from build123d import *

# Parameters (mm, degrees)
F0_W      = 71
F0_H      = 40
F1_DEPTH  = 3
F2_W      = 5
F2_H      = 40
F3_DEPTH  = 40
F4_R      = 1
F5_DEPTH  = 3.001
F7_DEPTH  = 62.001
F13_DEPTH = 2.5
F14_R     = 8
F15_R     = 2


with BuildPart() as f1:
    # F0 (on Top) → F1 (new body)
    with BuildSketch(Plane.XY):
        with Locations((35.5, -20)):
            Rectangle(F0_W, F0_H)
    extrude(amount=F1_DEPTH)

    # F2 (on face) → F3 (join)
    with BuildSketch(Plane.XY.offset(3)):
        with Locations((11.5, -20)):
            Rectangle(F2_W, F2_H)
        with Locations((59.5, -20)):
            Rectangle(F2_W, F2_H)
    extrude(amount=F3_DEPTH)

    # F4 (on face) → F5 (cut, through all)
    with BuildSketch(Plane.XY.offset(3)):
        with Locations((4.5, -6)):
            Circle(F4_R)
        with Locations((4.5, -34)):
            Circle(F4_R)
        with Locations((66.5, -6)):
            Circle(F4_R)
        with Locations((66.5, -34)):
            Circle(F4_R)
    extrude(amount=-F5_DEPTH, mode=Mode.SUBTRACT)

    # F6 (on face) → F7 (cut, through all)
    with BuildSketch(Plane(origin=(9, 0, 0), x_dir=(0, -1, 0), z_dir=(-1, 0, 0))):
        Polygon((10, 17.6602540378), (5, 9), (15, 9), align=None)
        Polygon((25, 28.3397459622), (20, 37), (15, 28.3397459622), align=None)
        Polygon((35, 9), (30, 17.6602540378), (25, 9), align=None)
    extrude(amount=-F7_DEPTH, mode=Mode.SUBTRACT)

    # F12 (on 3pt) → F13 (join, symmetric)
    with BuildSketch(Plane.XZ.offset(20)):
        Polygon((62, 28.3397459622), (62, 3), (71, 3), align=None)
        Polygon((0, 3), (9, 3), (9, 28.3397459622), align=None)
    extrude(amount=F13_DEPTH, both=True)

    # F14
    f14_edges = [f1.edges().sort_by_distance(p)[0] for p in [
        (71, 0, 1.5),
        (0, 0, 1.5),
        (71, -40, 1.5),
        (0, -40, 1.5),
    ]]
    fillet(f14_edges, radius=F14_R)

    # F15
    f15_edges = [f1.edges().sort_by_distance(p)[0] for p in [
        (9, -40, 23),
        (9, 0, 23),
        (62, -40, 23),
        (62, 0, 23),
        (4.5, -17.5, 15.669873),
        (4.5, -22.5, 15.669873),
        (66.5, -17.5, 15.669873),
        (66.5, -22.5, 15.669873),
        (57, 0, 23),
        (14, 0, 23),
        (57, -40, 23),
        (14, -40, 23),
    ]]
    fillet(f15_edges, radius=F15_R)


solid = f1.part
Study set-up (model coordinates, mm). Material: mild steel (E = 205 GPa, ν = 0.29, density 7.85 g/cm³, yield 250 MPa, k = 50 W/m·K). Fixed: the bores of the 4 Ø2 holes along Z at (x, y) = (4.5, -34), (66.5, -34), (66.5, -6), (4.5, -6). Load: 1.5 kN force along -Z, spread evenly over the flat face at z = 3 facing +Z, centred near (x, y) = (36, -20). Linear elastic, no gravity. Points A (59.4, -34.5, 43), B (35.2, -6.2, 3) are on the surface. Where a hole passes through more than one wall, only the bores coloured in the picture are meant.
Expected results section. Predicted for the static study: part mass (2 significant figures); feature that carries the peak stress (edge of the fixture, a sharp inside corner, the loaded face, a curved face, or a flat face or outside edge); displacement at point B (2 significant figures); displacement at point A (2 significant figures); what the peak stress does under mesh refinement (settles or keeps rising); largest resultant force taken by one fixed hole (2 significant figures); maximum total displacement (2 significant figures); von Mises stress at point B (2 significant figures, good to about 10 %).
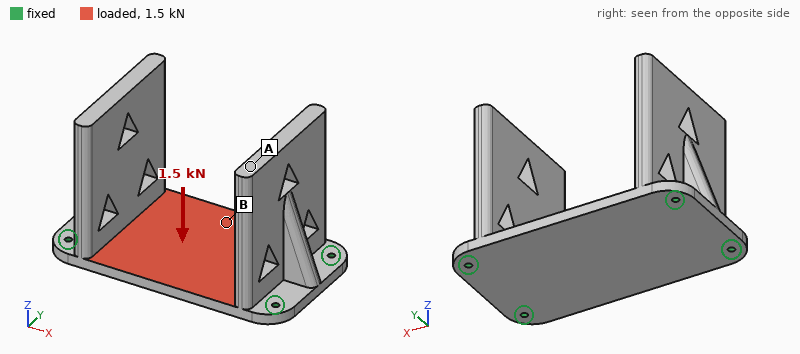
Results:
190 g
edge of the fixture
0.082 mm
0.13 mm
keeps rising
380 N
0.14 mm
92 MPa
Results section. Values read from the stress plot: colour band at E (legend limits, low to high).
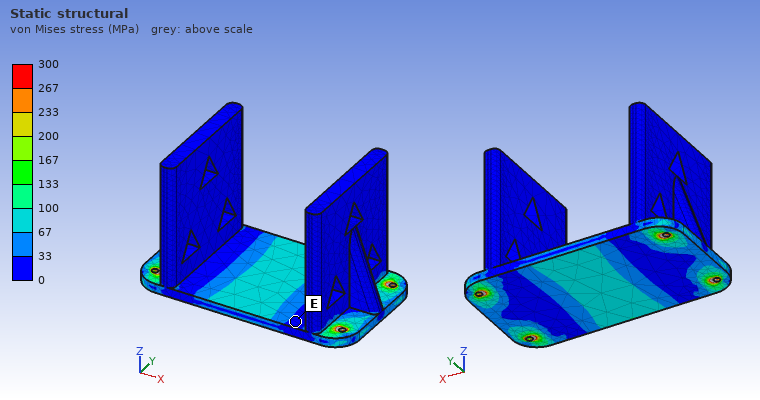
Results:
0 to 33 MPa
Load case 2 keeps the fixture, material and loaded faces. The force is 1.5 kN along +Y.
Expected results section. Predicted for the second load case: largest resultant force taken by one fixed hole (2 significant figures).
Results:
470 N
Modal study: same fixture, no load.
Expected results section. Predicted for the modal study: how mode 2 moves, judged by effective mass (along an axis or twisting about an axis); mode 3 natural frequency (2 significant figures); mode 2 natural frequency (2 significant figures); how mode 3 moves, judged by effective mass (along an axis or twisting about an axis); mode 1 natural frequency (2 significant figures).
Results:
along X
4000 Hz
1700 Hz
along Y
1300 Hz
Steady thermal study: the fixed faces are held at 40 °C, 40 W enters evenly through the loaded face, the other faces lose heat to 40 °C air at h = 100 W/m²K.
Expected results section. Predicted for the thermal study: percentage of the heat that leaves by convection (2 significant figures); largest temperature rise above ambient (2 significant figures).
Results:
50 %
52 K
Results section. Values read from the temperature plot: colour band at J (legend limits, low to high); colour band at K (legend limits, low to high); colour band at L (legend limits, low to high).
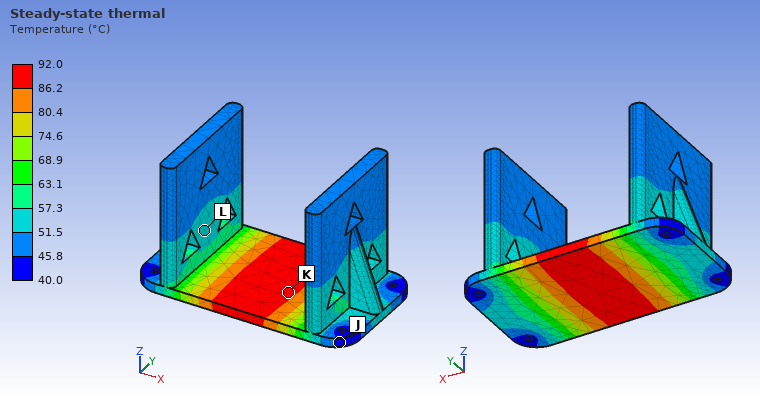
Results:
40.0 to 45.8 °C
86.2 to 92.0 °C
51.5 to 57.3 °C
